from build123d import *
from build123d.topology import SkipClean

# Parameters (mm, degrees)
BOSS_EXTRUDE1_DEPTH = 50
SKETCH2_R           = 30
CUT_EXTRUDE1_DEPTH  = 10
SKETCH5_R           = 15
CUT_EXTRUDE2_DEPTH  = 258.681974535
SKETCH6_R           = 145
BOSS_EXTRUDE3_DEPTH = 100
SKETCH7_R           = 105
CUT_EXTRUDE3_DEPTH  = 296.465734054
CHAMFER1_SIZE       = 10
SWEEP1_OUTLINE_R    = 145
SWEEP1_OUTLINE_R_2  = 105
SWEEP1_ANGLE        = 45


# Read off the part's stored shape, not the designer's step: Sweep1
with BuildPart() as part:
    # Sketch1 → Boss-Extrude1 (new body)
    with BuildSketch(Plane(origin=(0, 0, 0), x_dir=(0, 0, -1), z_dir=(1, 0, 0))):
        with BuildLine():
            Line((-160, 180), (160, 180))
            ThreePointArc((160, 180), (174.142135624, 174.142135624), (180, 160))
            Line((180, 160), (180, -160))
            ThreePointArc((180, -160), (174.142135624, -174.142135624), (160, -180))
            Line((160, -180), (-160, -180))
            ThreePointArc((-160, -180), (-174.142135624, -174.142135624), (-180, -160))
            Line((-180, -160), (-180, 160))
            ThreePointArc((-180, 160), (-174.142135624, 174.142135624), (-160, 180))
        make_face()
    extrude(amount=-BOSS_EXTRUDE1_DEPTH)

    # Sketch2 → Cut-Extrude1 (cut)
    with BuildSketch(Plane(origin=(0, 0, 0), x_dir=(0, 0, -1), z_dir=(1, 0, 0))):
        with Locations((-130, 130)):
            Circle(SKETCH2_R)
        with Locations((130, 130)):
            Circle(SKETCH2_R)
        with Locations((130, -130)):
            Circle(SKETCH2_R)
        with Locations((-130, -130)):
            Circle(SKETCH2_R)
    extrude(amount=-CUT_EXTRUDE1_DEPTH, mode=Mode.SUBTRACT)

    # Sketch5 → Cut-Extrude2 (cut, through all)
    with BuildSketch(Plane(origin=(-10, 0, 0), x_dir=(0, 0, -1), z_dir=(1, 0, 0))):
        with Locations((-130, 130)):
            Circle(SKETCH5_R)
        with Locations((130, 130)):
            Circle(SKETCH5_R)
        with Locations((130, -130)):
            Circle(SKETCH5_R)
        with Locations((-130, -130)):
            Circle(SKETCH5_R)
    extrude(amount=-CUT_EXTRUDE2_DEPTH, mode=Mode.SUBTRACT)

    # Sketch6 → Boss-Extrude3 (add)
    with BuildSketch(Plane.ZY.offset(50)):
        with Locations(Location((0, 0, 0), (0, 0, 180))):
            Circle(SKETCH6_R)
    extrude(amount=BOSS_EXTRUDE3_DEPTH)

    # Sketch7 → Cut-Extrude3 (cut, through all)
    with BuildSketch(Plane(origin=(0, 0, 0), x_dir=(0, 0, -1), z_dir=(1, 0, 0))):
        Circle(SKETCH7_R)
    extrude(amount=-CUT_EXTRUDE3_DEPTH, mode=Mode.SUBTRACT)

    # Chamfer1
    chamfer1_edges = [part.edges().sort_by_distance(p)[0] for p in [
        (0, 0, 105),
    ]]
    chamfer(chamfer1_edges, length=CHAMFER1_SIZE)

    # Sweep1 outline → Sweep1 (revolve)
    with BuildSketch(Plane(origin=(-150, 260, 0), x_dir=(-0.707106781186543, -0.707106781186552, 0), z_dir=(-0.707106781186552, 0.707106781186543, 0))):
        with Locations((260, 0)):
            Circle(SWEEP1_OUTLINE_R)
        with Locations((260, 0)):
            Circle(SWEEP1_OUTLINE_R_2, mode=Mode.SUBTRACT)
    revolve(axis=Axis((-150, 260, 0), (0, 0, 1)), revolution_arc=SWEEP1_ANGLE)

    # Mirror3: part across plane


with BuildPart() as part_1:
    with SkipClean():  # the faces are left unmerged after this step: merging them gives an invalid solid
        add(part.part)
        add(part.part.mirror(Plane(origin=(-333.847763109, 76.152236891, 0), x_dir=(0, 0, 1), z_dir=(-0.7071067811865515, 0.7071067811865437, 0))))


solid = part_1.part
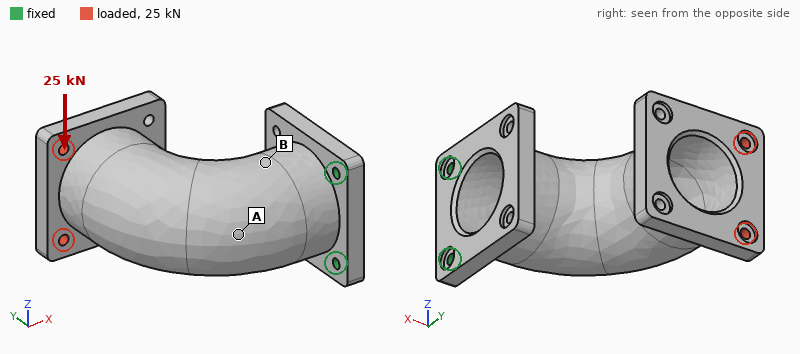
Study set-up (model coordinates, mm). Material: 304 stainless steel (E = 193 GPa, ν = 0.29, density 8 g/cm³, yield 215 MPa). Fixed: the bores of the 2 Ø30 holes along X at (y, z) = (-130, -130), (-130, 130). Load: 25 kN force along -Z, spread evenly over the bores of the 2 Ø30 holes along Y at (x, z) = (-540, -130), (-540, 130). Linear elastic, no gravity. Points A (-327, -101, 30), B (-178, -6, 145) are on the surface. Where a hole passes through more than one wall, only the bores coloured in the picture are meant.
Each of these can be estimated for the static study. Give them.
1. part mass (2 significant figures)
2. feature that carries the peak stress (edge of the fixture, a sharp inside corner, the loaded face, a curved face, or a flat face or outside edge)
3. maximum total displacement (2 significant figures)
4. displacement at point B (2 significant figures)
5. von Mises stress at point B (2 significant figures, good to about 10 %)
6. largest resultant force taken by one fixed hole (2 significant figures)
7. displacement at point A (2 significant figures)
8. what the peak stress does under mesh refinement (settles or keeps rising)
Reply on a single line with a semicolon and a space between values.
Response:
220 kg; edge of the fixture; 0.22 mm; 0.051 mm; 6.5 MPa; 71 kN; 0.061 mm; keeps rising
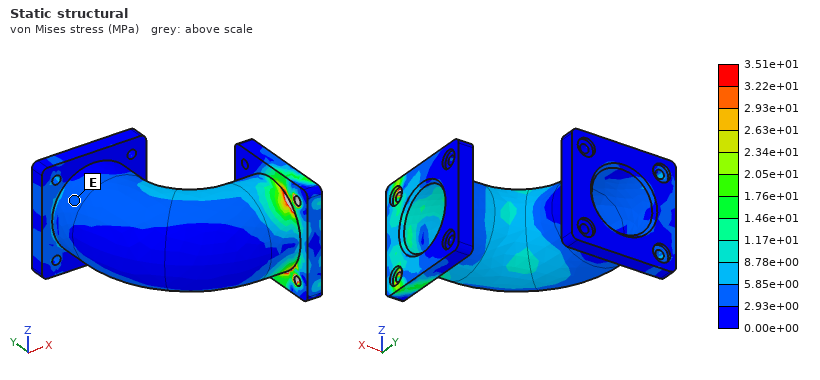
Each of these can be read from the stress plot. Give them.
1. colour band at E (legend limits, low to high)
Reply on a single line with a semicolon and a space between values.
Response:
2.93e+00 to 5.85e+00 MPa
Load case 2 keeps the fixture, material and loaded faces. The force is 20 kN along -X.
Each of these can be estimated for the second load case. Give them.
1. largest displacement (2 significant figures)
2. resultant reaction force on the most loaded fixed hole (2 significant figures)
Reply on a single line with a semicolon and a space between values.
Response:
1.1 mm; 10 kN
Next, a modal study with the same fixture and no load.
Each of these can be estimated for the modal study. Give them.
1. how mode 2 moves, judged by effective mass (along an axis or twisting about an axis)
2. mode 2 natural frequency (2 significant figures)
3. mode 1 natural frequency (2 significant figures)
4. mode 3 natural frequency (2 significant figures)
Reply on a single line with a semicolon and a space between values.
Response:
along Z; 210 Hz; 67 Hz; 530 Hz
